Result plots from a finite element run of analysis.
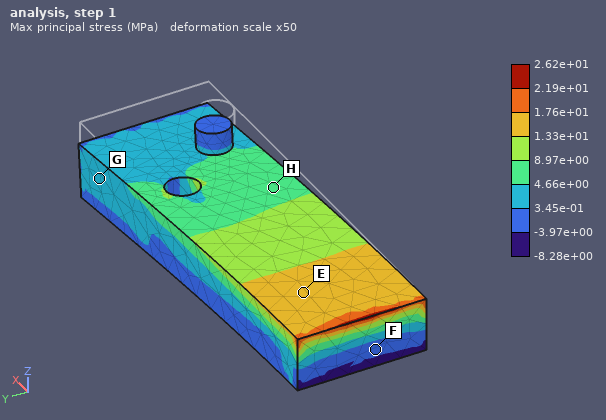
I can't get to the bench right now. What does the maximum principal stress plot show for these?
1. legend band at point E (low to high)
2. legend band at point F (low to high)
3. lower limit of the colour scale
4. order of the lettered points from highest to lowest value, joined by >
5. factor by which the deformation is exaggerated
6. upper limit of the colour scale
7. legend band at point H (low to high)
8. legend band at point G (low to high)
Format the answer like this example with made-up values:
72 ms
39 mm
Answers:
1.33e+01 to 1.76e+01 MPa
-3.97e+00 to 3.45e-01 MPa
-8.28e+00 MPa
E > H > G > F
50
2.62e+01 MPa
4.66e+00 to 8.97e+00 MPa
3.45e-01 to 4.66e+00 MPa
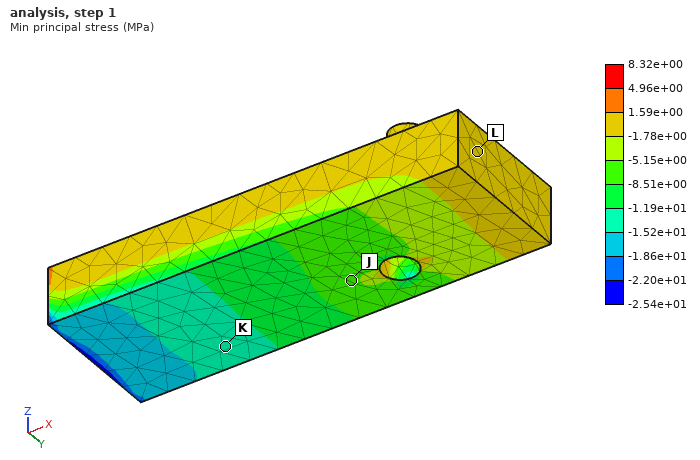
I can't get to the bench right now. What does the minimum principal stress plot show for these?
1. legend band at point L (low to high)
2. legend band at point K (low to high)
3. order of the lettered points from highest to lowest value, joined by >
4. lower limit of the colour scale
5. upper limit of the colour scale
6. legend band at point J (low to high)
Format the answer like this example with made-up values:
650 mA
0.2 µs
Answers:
-1.78e+00 to 1.59e+00 MPa
-1.52e+01 to -1.19e+01 MPa
L > J > K
-2.54e+01 MPa
8.32e+00 MPa
-8.51e+00 to -5.15e+00 MPa
